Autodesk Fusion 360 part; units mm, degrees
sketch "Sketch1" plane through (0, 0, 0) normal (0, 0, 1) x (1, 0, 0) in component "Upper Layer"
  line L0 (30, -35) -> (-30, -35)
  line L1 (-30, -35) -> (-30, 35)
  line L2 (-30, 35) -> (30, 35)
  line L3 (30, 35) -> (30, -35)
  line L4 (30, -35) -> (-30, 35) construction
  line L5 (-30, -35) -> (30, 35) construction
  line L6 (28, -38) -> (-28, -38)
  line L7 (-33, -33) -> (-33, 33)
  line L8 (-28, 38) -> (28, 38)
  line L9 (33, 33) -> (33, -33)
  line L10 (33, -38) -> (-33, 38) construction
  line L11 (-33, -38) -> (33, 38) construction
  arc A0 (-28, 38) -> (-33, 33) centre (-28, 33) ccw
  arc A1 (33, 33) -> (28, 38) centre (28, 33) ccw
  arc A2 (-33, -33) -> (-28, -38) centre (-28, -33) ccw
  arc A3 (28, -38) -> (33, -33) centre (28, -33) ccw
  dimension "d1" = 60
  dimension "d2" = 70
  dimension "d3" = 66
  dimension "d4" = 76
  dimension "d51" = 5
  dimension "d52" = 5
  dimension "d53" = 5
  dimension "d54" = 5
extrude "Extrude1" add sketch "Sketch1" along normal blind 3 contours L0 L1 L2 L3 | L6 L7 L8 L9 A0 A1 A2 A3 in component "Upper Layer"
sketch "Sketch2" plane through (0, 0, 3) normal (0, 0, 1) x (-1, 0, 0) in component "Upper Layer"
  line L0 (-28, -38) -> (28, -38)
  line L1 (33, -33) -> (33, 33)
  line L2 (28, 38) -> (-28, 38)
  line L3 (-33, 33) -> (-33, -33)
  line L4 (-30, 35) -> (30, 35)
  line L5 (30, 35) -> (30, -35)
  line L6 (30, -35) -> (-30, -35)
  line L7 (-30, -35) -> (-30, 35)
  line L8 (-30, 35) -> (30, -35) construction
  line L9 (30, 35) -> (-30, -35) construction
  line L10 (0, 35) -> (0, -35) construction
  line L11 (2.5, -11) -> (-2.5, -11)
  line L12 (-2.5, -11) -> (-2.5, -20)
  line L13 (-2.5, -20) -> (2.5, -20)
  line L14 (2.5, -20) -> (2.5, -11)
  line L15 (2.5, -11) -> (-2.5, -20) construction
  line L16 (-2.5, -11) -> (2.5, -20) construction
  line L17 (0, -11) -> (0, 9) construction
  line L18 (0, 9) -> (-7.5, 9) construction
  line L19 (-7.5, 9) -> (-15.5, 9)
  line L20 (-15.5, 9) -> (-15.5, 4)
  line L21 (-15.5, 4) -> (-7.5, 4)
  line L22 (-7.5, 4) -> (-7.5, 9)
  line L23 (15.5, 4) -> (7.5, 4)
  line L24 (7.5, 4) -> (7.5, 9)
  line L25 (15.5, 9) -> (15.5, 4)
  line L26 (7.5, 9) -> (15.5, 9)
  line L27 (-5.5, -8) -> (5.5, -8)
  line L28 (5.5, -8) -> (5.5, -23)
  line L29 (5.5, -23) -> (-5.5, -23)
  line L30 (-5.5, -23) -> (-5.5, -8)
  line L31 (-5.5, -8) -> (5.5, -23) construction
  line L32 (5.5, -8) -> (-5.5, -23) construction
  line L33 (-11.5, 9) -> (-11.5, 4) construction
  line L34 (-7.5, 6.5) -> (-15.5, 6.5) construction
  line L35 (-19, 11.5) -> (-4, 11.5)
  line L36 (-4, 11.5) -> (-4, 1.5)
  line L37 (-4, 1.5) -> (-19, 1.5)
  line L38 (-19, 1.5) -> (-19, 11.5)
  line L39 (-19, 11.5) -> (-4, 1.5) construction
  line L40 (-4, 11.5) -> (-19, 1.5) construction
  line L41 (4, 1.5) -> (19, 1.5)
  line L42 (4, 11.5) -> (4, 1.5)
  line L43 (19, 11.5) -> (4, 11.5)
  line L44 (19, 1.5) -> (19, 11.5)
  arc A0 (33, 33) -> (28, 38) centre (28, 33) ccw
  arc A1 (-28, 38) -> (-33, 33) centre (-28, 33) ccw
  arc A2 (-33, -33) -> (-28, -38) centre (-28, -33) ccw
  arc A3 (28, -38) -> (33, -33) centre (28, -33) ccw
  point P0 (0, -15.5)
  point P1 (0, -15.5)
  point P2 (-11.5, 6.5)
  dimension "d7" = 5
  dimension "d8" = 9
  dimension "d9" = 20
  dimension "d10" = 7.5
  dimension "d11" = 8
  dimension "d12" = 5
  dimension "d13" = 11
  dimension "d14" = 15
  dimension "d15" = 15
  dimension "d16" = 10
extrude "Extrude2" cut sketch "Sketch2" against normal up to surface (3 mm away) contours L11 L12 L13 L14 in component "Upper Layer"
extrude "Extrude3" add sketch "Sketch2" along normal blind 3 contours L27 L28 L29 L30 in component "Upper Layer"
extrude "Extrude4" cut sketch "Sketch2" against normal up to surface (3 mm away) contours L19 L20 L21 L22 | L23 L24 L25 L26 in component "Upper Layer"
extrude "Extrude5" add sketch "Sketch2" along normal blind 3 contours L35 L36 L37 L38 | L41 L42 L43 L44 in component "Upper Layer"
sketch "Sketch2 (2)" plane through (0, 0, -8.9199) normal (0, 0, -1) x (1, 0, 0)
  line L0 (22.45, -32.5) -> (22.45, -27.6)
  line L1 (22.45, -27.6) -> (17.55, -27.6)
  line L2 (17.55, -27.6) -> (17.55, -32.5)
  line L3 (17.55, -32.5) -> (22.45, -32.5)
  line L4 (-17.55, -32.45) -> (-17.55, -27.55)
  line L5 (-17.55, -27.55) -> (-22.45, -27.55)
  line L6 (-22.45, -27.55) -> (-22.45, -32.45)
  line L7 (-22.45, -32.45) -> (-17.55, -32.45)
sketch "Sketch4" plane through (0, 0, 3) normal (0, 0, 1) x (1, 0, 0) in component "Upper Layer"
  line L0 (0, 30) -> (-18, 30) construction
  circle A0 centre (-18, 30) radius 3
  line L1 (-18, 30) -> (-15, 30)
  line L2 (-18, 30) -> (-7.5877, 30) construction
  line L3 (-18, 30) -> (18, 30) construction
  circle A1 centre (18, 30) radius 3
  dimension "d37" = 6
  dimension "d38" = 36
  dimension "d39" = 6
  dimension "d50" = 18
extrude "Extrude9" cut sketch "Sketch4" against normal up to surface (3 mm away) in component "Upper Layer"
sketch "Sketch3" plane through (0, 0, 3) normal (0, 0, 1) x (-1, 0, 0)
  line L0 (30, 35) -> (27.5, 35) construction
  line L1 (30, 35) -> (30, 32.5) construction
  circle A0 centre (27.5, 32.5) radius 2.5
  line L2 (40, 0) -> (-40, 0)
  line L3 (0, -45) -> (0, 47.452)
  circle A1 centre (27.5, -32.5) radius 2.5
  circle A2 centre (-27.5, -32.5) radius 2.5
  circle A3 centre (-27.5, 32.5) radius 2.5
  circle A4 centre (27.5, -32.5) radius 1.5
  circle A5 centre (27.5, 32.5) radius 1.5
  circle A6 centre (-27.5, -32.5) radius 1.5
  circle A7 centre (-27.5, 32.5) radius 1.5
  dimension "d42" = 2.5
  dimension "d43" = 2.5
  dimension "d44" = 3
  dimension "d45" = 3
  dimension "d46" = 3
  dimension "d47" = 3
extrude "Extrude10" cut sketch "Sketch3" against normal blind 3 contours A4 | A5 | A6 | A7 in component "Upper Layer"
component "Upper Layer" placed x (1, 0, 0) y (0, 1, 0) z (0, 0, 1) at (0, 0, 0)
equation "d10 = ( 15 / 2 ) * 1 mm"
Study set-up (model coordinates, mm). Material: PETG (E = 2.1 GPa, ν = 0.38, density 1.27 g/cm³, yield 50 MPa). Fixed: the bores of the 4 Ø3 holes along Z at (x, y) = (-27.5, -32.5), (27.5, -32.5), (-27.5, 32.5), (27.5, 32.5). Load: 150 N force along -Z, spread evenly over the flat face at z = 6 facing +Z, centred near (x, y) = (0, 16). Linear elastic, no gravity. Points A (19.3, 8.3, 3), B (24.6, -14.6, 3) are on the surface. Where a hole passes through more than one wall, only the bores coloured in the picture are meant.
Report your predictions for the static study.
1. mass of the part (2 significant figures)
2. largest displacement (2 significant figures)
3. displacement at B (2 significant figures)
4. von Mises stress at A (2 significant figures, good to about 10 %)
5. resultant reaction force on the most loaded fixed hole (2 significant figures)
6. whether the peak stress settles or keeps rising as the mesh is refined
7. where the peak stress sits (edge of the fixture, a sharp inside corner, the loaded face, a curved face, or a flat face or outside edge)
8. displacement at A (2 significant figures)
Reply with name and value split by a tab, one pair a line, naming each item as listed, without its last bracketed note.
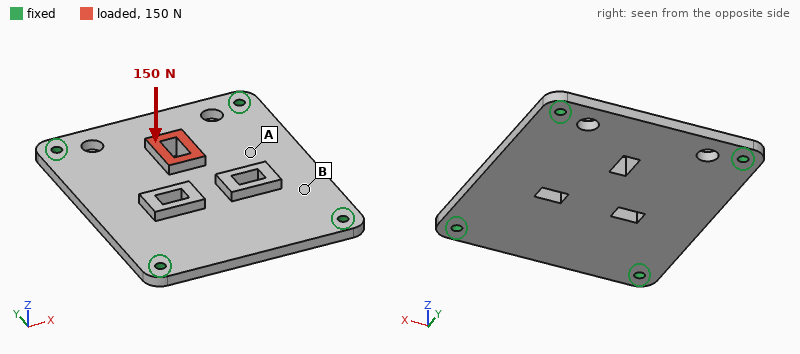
mass of the part	20 g
largest displacement	1.1 mm
displacement at B	0.32 mm
von Mises stress at A	6.8 MPa
resultant reaction force on the most loaded fixed hole	59 N
whether the peak stress settles or keeps rising as the mesh is refined	keeps rising
where the peak stress sits	edge of the fixture
displacement at A	0.68 mm
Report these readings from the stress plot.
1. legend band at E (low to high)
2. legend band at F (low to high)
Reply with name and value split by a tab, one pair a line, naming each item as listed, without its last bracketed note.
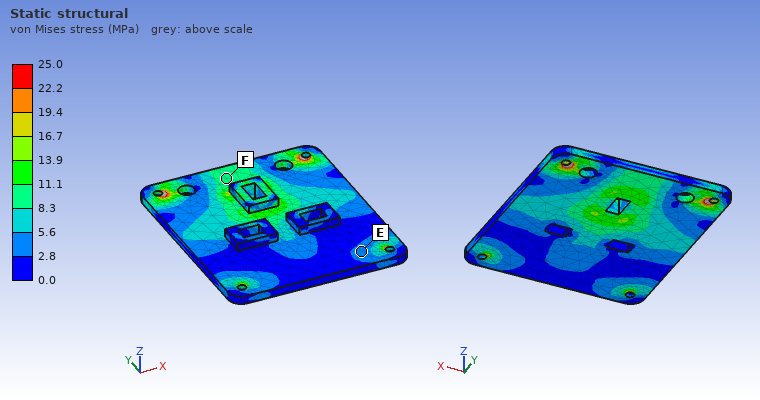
legend band at E	2.8 to 5.6 MPa
legend band at F	8.3 to 11.1 MPa
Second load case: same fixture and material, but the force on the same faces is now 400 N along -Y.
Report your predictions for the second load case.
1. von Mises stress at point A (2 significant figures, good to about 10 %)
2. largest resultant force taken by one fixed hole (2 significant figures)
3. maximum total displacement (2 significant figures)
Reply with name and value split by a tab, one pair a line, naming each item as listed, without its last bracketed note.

von Mises stress at point A	5.9 MPa
largest resultant force taken by one fixed hole	110 N
maximum total displacement	0.50 mm
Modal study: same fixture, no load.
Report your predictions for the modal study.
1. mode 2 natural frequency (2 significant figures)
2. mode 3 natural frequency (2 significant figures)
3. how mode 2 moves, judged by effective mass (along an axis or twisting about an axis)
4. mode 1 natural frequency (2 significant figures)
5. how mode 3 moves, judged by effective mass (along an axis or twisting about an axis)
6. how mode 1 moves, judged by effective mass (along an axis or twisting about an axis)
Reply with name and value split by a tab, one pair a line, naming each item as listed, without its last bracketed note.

mode 2 natural frequency	1100 Hz
mode 3 natural frequency	1300 Hz
how mode 2 moves, judged by effective mass	twisting about Y
mode 1 natural frequency	680 Hz
how mode 3 moves, judged by effective mass	twisting about X
how mode 1 moves, judged by effective mass	along Z
